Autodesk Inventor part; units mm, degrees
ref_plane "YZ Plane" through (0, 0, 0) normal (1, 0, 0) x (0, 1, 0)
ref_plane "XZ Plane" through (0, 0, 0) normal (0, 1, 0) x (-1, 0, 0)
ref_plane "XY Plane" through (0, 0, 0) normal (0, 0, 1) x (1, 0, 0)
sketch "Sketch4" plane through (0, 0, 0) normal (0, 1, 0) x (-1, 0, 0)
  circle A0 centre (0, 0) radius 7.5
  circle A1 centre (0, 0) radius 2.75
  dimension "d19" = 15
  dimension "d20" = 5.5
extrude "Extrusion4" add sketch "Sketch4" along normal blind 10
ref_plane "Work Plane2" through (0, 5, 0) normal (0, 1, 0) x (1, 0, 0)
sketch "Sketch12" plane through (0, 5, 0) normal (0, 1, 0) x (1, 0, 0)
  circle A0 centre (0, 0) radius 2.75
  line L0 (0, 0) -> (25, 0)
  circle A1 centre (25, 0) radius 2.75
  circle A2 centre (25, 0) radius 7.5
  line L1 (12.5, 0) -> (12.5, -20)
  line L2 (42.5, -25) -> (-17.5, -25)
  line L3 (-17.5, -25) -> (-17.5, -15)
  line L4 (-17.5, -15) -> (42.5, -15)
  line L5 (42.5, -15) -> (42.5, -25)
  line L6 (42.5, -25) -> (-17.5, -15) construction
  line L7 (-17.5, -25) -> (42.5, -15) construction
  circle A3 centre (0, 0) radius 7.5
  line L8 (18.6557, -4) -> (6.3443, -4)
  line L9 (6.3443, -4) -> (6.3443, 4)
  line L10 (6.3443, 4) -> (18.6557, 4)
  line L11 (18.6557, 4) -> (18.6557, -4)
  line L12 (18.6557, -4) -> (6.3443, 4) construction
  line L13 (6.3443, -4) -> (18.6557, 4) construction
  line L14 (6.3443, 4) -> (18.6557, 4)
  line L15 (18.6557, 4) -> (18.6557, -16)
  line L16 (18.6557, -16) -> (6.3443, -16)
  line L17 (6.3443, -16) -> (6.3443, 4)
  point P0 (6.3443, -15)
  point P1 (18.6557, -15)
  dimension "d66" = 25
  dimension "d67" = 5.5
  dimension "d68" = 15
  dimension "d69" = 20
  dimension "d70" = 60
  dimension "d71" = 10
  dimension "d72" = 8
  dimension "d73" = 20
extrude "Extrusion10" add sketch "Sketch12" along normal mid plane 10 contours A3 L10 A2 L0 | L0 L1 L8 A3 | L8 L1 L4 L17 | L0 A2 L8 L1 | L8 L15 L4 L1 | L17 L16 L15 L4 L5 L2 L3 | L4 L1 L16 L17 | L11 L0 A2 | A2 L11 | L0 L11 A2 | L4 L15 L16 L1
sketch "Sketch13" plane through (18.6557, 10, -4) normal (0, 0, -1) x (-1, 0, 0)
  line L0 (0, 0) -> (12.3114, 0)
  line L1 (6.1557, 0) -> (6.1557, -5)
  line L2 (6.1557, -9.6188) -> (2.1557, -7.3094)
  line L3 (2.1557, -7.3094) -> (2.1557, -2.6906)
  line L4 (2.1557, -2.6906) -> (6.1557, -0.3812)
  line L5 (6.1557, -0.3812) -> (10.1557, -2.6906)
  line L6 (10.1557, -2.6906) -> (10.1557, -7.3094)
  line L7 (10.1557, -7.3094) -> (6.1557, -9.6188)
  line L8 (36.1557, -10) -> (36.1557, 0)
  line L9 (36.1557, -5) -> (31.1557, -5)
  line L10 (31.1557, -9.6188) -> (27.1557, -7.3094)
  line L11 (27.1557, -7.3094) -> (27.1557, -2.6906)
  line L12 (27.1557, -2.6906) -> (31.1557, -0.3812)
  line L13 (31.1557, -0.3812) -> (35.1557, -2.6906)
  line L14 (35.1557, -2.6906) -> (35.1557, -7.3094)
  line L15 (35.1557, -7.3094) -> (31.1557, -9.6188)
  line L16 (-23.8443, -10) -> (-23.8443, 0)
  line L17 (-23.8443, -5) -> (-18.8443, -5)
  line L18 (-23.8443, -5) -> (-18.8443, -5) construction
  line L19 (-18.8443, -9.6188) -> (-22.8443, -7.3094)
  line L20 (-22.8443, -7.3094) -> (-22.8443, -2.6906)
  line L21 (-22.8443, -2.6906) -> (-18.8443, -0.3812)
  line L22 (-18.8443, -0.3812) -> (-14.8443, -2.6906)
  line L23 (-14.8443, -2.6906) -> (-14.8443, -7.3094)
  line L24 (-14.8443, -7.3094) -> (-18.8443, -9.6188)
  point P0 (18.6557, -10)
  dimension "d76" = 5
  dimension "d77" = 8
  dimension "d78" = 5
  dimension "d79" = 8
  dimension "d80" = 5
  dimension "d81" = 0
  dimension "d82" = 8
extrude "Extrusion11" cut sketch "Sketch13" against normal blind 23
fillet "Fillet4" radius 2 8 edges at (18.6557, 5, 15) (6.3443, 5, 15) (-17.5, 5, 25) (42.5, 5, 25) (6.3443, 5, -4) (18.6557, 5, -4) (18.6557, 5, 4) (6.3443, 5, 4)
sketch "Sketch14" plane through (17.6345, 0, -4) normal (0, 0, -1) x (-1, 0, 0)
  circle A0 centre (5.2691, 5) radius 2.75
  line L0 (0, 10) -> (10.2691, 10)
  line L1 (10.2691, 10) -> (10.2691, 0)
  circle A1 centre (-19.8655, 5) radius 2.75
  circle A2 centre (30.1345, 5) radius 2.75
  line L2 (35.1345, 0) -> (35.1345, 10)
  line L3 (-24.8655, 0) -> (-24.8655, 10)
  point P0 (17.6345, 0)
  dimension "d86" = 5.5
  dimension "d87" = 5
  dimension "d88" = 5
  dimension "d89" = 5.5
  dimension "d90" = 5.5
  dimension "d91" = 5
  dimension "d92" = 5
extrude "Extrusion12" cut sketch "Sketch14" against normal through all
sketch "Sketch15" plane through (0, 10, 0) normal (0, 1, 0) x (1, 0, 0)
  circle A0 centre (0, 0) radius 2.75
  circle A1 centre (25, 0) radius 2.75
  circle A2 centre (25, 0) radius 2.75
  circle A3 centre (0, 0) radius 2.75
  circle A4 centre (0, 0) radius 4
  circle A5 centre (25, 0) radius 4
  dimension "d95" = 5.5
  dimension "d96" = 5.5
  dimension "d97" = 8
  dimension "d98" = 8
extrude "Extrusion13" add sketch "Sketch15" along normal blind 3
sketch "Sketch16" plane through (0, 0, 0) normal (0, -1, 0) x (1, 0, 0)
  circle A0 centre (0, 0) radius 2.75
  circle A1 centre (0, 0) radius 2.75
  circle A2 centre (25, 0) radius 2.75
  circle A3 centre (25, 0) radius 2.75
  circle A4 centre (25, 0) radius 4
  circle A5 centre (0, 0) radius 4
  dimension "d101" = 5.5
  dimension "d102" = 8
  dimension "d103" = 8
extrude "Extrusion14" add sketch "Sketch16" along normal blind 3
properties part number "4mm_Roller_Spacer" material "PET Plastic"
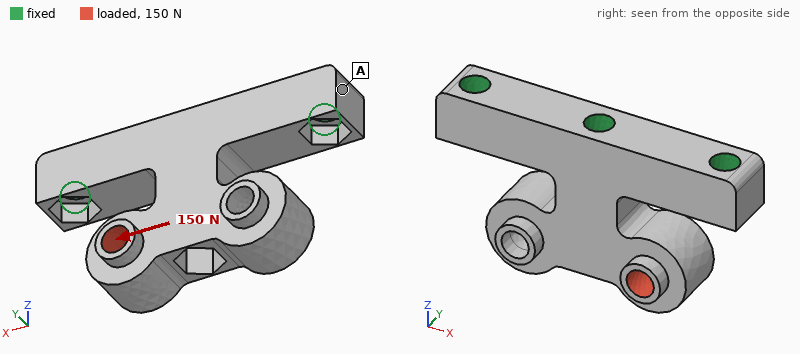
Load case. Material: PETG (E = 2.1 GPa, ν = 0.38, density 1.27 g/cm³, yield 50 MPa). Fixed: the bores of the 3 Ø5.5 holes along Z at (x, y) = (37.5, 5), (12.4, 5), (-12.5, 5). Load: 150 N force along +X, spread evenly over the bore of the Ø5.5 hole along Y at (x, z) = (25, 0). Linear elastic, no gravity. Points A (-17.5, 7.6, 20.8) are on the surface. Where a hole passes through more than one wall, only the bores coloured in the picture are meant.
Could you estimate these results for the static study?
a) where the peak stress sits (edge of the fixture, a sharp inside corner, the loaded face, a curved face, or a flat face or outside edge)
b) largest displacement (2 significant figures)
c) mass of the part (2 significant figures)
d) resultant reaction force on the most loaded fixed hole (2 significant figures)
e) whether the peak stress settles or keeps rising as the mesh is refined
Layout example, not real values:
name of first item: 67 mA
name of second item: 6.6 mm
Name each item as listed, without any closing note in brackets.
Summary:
where the peak stress sits: a sharp inside corner
largest displacement: 0.41 mm
mass of the part: 12 g
resultant reaction force on the most loaded fixed hole: 88 N
whether the peak stress settles or keeps rising as the mesh is refined: keeps rising
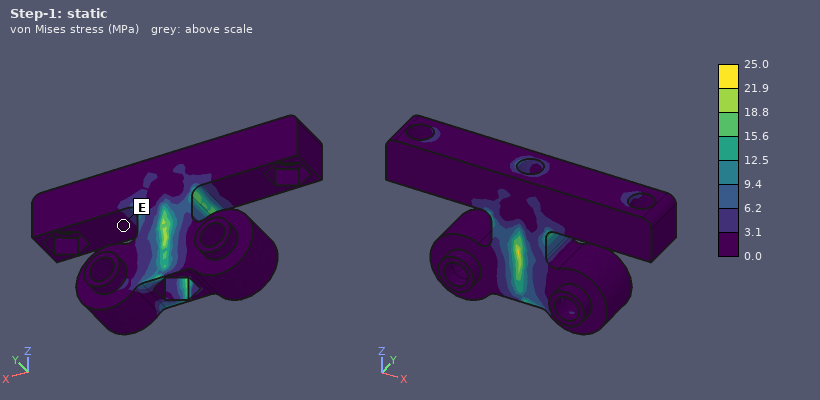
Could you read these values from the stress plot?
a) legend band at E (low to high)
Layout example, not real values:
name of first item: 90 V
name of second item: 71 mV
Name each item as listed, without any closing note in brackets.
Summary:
legend band at E: 0.0 to 3.1 MPa
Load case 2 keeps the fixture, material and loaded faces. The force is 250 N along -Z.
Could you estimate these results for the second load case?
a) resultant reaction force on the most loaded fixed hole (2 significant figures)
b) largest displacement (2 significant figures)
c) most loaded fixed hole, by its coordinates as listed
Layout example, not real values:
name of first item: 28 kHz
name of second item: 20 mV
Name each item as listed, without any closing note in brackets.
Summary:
resultant reaction force on the most loaded fixed hole: 250 N
largest displacement: 0.75 mm
most loaded fixed hole, by its coordinates as listed: (12.4, 5)
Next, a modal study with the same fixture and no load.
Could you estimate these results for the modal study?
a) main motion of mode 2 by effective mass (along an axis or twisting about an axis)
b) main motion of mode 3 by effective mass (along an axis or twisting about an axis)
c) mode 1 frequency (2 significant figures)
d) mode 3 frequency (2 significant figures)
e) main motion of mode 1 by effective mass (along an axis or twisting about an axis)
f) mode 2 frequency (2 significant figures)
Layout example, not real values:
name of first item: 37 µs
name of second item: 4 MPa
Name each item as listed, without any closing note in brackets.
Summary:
main motion of mode 2 by effective mass: along X
main motion of mode 3 by effective mass: twisting about Z
mode 1 frequency: 1300 Hz
mode 3 frequency: 1500 Hz
main motion of mode 1 by effective mass: along Y
mode 2 frequency: 1400 Hz
